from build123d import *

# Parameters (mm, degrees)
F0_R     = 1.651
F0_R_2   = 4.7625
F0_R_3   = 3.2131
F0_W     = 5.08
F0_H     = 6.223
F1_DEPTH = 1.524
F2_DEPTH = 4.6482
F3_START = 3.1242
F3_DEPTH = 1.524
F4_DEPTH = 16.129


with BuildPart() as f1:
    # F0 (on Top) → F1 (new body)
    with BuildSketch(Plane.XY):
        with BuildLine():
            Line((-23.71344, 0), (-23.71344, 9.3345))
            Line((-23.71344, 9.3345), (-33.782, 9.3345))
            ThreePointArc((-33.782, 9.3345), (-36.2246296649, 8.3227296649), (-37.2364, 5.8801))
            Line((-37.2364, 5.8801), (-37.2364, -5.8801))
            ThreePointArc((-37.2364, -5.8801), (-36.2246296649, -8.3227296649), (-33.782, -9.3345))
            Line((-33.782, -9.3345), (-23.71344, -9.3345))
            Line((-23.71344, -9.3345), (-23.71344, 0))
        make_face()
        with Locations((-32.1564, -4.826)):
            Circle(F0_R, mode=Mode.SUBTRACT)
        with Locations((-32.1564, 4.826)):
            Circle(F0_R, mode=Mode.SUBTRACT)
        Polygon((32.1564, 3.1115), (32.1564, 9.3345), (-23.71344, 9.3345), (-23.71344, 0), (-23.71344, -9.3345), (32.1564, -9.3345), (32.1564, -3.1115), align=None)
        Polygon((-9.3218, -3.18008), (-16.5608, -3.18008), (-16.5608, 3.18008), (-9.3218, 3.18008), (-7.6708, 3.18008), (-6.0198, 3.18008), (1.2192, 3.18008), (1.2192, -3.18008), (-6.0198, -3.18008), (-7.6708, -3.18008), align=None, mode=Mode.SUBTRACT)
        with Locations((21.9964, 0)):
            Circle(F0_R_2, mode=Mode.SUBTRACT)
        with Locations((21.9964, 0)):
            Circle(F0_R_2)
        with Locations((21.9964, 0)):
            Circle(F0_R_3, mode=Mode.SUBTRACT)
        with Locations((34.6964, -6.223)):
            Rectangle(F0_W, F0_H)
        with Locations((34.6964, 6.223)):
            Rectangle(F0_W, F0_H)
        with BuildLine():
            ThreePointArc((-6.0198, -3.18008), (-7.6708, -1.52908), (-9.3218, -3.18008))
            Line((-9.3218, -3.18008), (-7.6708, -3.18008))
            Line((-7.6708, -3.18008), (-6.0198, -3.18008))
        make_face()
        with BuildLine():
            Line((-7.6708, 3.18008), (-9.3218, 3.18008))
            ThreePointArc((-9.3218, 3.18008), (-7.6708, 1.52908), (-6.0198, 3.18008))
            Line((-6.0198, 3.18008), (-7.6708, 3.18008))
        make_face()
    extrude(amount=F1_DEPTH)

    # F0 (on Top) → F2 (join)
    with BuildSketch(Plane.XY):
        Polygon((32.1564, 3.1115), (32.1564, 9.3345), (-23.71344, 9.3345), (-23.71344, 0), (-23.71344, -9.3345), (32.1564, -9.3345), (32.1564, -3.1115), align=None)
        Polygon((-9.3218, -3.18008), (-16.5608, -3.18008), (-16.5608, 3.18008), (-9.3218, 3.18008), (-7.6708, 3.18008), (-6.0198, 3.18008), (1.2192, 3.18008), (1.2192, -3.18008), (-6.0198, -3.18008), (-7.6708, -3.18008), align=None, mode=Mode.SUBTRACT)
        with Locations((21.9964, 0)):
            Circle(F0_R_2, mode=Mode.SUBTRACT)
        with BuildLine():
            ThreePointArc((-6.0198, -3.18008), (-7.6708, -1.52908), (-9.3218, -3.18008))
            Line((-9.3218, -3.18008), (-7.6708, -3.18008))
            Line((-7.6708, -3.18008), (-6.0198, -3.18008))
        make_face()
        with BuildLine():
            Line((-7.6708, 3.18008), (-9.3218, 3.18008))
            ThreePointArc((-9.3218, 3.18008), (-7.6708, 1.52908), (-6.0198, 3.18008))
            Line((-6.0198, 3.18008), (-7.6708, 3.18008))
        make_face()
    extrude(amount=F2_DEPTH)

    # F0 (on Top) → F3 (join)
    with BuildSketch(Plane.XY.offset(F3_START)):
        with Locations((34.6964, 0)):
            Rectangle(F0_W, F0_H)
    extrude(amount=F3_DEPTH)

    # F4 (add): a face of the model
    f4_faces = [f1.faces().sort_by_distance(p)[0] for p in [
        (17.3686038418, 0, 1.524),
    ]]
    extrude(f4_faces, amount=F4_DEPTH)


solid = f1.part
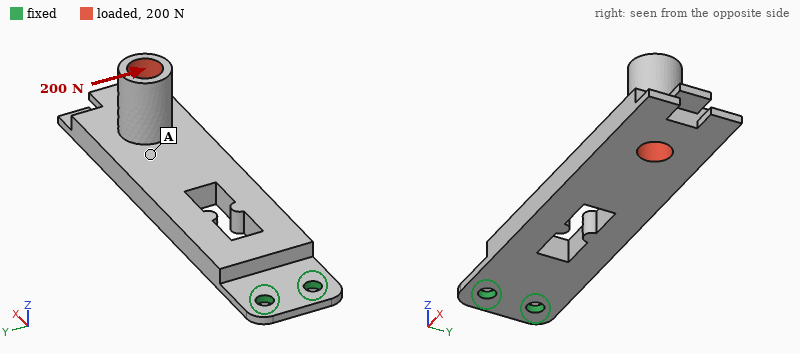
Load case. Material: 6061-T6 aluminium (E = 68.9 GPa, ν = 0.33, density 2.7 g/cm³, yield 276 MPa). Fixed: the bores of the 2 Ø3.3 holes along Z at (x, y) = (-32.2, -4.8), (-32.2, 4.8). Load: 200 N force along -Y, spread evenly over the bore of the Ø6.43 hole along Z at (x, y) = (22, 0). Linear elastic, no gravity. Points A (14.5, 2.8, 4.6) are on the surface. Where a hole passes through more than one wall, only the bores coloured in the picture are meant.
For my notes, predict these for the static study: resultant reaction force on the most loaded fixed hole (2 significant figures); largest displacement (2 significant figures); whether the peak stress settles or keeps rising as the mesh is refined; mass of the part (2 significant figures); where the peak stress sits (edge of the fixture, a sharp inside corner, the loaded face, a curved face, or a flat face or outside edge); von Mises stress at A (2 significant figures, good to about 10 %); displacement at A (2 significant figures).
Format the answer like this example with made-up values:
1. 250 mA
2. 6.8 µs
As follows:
1. 940 N
2. 0.34 mm
3. keeps rising
4. 14 g
5. edge of the fixture
6. 24 MPa
7. 0.16 mm
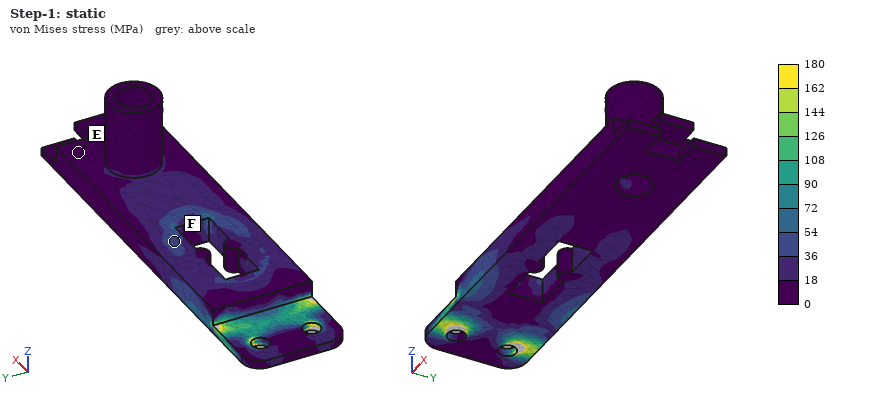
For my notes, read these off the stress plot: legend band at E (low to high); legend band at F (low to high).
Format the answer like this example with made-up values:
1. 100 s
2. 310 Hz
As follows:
1. 0 to 18 MPa
2. 36 to 54 MPa
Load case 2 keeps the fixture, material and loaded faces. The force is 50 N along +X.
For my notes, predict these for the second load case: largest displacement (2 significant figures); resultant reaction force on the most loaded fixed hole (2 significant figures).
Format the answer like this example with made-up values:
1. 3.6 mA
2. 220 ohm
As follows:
1. 0.58 mm
2. 25 N
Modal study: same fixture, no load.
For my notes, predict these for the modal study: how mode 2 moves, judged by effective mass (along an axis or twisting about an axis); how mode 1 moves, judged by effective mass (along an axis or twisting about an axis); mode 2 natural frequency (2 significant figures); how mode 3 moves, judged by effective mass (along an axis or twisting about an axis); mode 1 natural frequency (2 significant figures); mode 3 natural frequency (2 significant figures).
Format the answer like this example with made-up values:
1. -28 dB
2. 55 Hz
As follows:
1. along Y
2. along Z
3. 1900 Hz
4. twisting about X
5. 240 Hz
6. 2600 Hz
